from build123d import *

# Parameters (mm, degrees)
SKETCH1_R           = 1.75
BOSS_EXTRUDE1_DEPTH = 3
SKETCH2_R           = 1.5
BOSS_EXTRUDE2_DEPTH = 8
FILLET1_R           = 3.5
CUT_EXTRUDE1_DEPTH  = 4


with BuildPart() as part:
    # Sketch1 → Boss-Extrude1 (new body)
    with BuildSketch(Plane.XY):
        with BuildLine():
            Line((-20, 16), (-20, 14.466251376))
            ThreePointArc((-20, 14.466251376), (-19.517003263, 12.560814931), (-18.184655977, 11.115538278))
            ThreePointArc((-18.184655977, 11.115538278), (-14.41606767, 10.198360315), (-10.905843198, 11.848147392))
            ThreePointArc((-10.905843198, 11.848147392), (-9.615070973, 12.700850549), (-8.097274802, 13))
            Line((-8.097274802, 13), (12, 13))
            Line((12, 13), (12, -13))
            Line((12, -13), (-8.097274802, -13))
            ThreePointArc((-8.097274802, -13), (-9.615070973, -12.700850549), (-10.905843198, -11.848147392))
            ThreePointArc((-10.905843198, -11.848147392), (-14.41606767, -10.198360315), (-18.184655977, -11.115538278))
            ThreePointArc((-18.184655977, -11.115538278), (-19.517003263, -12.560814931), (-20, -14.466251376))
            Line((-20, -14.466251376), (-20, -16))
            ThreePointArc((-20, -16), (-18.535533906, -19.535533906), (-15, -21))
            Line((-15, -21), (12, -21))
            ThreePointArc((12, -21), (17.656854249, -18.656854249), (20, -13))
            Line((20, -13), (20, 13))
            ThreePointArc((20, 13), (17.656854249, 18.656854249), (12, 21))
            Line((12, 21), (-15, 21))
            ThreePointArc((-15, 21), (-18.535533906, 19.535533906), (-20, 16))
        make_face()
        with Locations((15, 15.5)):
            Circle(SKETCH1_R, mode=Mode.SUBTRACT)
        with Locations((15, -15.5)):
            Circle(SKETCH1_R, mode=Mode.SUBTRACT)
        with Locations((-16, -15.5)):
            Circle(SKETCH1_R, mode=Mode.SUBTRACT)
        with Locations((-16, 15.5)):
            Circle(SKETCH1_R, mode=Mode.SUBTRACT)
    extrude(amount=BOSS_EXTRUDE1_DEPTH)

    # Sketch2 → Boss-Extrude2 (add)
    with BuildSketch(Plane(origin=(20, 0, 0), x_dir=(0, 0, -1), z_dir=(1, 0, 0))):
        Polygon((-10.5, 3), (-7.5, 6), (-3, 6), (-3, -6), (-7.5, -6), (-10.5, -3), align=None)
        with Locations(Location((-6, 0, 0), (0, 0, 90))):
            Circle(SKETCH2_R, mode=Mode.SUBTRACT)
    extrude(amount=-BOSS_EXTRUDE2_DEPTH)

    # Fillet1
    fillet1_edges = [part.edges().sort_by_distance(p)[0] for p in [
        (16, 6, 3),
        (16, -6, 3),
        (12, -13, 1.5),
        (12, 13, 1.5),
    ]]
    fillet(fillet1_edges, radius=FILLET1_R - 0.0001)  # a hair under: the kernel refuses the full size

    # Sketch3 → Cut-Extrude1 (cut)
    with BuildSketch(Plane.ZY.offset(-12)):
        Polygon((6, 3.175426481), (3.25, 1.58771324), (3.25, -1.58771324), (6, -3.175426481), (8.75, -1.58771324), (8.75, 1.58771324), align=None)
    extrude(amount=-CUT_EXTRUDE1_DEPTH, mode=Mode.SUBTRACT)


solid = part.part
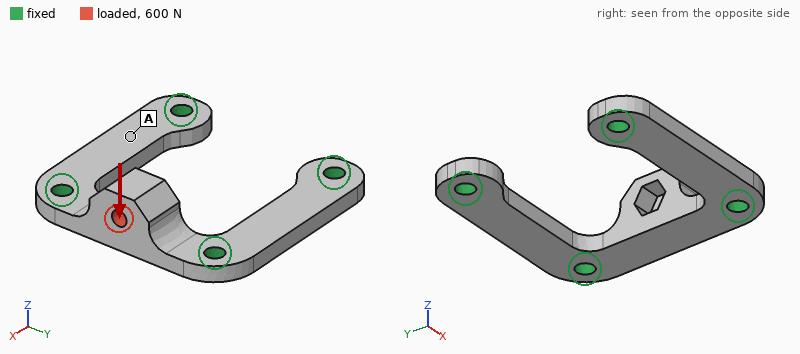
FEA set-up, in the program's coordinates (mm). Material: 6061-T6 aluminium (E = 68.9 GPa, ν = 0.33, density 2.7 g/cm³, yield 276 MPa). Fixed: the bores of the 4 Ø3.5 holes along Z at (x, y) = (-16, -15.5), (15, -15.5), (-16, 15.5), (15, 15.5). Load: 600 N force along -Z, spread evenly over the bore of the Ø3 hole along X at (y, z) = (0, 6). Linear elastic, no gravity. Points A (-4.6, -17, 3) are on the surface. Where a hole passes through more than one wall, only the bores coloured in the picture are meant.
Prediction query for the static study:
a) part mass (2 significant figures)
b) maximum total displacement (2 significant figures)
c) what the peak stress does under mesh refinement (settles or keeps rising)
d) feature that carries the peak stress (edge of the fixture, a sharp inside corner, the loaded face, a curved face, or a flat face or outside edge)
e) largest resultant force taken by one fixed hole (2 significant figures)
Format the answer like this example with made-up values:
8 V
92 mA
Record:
8.1 g
45 µm
keeps rising
edge of the fixture
360 N
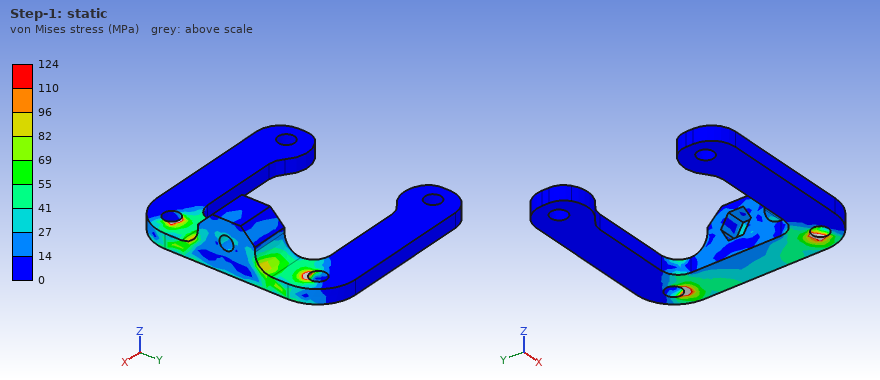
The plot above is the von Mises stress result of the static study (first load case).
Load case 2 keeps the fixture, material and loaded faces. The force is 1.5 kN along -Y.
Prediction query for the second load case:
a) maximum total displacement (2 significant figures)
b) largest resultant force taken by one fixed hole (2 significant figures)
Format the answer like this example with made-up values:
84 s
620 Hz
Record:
19 µm
810 N
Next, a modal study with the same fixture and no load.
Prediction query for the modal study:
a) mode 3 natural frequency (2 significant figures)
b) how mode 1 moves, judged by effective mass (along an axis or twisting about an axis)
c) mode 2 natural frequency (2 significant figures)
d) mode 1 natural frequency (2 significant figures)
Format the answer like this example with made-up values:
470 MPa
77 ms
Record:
18 kHz
along X
18 kHz
13 kHz
